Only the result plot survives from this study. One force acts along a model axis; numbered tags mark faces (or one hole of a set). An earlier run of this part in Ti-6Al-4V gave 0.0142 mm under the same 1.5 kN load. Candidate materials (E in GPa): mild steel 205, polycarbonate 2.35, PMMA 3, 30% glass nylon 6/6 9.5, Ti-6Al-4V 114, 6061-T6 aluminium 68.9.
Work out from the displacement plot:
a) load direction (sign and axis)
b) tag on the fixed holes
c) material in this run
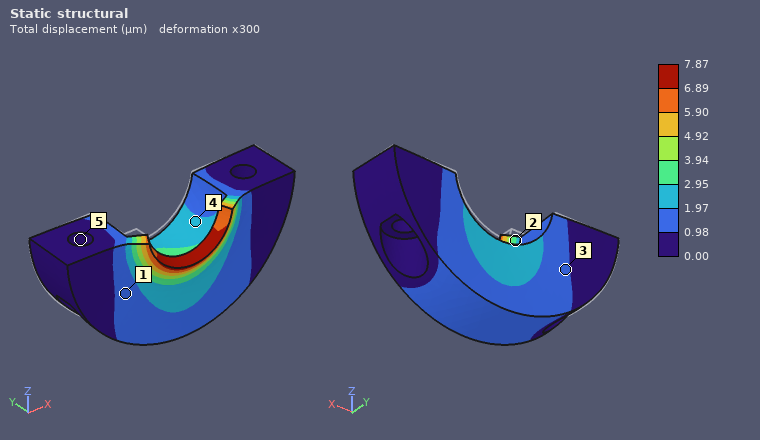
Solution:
-Y
5
mild steel
